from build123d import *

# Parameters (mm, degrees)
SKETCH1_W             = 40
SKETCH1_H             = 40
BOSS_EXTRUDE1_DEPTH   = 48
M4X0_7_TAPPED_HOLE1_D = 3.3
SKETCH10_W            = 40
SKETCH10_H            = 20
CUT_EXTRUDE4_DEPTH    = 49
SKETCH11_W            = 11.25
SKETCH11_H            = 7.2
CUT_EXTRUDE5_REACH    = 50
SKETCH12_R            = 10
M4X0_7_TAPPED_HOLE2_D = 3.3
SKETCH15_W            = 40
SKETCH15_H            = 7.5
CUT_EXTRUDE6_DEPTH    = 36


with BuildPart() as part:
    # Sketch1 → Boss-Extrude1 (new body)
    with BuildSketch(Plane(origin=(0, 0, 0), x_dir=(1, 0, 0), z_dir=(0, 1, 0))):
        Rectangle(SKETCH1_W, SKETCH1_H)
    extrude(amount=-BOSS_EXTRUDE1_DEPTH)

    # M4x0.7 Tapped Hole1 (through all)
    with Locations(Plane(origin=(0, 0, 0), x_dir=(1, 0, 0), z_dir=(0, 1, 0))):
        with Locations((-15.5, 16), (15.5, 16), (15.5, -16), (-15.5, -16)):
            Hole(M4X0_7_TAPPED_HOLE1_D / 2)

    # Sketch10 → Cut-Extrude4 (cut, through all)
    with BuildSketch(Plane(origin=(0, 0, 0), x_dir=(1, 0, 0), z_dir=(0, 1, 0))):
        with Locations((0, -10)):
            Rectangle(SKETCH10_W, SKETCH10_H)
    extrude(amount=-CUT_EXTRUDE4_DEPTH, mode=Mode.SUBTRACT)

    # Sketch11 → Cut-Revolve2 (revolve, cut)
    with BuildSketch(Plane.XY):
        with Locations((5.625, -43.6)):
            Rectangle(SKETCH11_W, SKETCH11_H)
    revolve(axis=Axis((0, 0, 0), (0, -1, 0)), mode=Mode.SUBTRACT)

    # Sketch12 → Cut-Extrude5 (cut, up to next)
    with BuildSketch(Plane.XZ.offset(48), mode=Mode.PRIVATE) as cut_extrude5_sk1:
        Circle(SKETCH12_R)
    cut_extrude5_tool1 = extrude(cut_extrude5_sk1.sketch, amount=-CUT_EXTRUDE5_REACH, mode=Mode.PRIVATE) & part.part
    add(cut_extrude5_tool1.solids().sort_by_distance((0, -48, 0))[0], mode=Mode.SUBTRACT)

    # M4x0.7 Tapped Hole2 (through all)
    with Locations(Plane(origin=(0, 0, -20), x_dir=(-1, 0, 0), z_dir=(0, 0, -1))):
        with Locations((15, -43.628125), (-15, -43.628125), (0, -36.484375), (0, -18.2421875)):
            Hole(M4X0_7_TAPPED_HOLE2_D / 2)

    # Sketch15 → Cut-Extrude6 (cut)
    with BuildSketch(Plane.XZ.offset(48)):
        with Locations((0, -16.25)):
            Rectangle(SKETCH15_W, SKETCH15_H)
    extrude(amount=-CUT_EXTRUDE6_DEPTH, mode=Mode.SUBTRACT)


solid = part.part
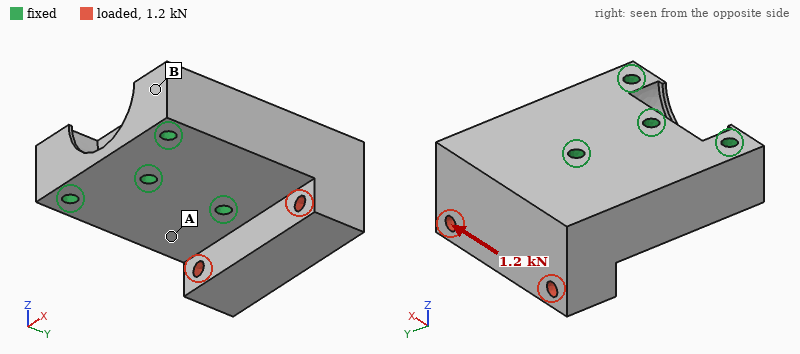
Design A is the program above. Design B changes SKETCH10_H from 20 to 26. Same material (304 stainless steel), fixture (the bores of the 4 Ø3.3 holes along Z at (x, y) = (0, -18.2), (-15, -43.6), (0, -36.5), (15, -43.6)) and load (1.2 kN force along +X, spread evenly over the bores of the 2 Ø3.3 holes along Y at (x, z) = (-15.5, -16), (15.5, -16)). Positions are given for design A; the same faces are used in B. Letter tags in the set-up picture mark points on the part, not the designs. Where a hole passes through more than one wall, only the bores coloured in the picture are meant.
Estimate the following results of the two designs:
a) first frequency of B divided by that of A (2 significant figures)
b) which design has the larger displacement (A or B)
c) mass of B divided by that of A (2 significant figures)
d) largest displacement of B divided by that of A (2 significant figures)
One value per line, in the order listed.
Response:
0.82
B
0.80
1.4
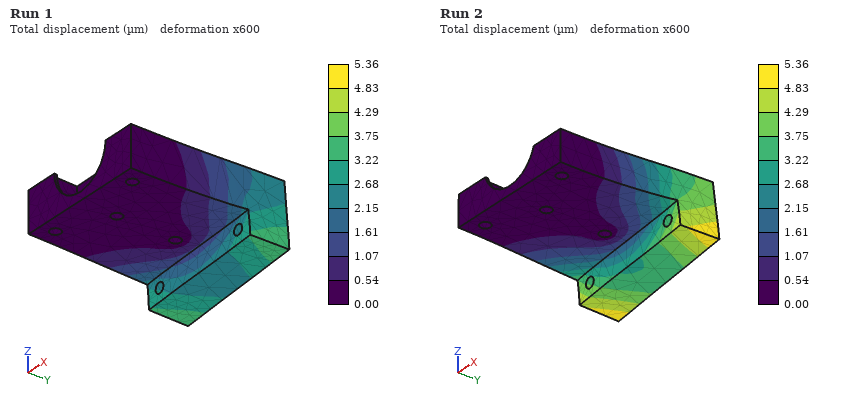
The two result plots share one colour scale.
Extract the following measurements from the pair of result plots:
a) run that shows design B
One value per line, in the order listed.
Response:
Run 2
